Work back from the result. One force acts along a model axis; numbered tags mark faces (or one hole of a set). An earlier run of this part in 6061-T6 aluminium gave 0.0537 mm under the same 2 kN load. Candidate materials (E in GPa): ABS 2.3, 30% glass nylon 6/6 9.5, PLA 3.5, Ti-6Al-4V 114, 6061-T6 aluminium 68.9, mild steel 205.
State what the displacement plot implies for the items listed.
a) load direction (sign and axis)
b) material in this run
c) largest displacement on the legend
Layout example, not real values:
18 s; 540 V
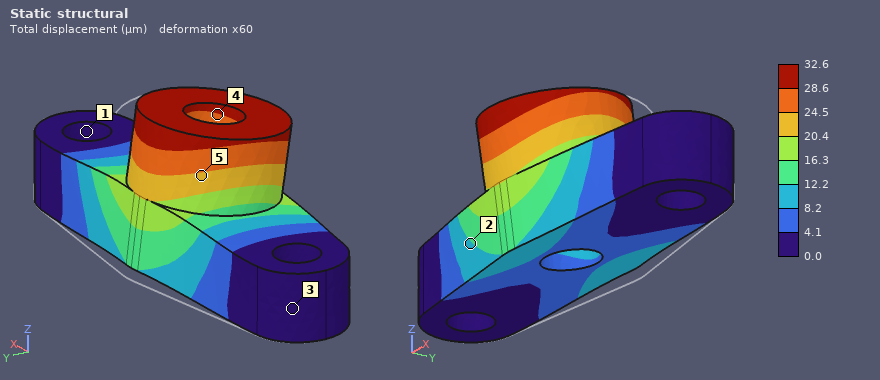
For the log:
-Y; Ti-6Al-4V; 32.6 µm
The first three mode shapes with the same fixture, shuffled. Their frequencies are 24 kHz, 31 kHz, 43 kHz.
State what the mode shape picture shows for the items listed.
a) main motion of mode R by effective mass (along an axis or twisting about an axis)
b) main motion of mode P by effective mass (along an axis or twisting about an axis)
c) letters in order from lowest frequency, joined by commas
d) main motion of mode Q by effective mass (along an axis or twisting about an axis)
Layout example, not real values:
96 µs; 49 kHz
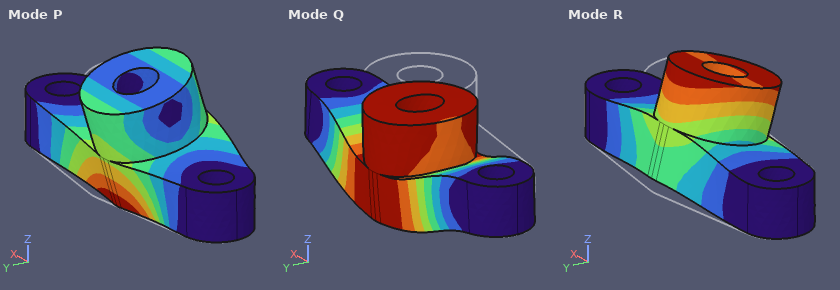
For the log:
along Y; along Y; R, Q, P; along Z
